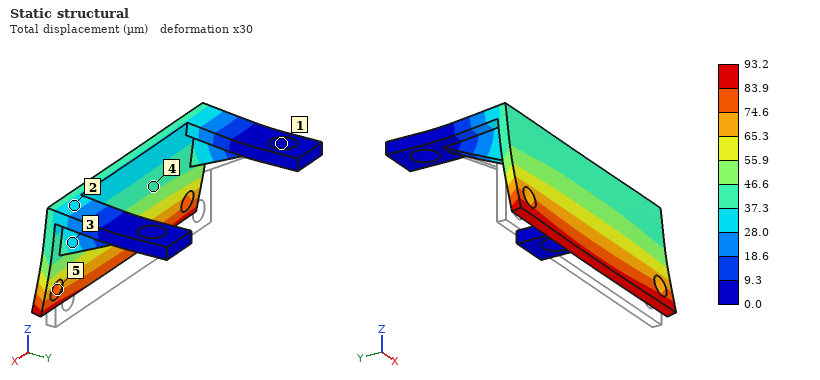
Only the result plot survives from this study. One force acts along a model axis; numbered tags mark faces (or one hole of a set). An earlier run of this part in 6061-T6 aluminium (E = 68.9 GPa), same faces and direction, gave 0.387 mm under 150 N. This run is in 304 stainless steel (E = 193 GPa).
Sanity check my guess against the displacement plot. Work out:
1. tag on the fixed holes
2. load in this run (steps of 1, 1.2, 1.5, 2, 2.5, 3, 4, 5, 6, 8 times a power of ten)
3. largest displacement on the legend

1
100 N
93.2 µm
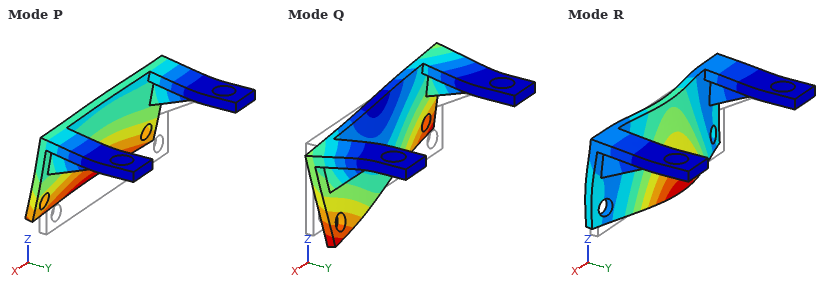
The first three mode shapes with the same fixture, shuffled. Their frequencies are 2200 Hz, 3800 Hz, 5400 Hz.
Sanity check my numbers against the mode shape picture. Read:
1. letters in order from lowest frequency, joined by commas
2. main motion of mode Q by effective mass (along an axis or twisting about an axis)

P, Q, R
along X
